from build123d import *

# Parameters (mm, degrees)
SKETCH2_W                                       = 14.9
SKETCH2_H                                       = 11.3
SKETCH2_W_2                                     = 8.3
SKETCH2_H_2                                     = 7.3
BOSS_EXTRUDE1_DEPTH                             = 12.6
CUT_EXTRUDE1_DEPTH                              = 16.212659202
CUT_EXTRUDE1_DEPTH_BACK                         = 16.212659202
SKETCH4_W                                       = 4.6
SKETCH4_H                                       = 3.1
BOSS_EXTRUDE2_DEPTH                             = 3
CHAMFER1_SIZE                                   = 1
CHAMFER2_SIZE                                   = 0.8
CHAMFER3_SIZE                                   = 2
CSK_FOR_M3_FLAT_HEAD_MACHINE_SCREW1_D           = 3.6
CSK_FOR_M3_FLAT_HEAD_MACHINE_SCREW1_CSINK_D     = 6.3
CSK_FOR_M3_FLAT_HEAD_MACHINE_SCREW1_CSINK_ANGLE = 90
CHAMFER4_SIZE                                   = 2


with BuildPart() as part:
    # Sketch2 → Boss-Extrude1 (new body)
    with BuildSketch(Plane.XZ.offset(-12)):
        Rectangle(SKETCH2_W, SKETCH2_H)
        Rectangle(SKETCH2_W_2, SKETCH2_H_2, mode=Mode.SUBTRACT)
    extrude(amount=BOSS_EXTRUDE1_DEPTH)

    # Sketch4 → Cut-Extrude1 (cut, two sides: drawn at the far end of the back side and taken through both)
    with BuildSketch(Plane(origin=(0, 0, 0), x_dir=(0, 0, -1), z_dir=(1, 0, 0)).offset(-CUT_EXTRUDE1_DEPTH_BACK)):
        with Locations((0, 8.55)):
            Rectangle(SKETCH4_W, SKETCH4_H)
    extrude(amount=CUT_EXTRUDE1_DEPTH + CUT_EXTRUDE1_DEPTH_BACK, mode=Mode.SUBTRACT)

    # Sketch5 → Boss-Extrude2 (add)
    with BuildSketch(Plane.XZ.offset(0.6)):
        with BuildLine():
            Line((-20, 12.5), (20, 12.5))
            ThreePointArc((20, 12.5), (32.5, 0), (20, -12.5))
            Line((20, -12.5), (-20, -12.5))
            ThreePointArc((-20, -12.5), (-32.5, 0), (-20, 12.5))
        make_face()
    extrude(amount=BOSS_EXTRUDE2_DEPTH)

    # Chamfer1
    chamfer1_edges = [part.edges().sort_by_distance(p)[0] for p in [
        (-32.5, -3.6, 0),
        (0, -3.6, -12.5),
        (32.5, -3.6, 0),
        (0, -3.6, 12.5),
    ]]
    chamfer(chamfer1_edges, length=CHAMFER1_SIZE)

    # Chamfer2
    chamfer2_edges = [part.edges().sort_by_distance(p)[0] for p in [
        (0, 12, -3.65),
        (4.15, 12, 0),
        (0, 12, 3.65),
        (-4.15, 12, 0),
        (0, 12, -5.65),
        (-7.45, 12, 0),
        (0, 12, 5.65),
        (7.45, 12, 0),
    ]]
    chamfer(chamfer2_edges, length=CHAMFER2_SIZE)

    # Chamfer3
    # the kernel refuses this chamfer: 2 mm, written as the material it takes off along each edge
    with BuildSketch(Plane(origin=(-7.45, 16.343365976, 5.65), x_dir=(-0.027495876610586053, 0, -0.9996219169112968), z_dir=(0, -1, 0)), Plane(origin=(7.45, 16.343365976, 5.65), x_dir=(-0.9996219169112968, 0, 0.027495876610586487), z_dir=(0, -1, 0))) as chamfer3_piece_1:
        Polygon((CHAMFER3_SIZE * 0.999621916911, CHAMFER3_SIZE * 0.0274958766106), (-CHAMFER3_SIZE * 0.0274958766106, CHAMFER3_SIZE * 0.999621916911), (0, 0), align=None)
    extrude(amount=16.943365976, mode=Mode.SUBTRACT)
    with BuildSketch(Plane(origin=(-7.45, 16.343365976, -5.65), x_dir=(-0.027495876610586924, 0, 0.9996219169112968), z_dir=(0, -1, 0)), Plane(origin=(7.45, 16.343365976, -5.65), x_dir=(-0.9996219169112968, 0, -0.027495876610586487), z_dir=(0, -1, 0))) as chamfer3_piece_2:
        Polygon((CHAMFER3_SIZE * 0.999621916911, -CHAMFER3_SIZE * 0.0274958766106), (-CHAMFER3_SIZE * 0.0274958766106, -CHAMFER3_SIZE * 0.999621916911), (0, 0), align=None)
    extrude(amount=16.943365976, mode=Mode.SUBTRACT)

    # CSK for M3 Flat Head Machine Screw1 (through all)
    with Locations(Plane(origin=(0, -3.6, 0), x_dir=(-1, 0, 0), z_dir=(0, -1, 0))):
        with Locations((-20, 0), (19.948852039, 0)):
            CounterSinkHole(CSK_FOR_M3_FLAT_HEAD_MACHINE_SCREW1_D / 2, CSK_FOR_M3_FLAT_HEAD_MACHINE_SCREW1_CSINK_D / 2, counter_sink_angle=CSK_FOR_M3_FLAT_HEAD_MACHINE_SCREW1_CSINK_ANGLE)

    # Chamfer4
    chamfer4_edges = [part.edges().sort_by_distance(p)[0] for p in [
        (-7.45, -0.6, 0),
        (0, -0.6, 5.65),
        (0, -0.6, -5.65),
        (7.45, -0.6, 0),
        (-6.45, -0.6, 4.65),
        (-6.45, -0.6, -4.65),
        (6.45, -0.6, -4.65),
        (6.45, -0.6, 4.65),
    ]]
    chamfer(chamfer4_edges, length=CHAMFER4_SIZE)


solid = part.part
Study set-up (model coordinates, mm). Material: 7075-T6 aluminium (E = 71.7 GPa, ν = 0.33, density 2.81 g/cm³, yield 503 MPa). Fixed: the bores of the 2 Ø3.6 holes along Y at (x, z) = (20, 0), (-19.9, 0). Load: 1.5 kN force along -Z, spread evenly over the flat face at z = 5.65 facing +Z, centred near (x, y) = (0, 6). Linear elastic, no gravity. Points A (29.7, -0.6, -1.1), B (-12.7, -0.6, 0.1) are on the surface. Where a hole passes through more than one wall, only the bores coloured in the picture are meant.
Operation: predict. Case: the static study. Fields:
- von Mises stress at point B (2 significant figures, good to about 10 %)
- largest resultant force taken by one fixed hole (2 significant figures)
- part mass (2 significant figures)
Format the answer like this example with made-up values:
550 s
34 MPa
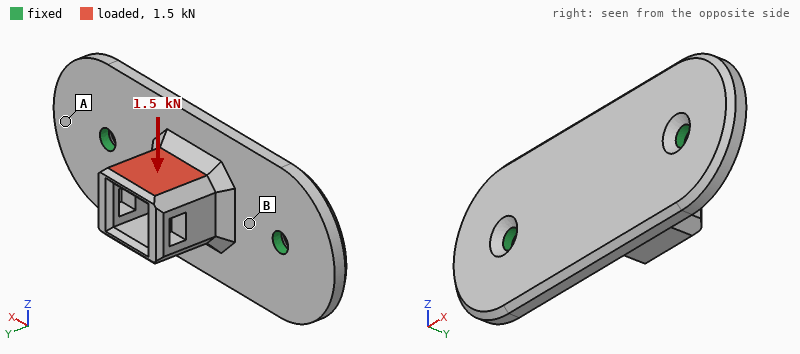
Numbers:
150 MPa
750 N
16 g
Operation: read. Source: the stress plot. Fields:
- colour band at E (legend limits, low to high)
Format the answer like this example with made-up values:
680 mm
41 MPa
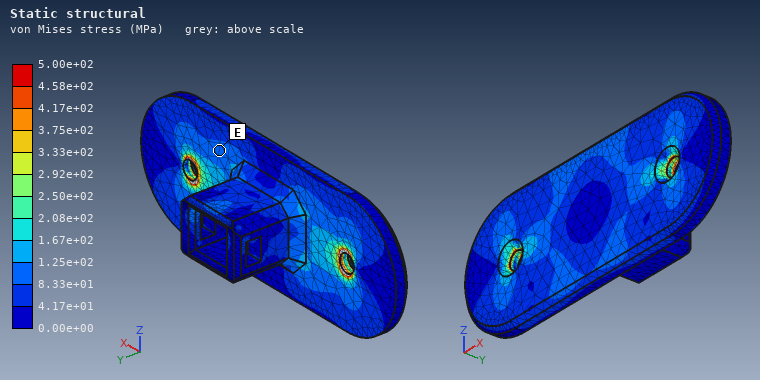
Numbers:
8.33e+01 to 1.25e+02 MPa
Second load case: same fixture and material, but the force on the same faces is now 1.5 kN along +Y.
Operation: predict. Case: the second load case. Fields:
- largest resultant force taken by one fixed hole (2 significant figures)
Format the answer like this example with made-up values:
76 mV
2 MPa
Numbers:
770 N
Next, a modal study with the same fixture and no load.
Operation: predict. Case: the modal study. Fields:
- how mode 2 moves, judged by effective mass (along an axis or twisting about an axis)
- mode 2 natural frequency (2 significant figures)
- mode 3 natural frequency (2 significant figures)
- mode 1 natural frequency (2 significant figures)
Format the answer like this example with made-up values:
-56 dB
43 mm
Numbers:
along Y
7100 Hz
13 kHz
5500 Hz
